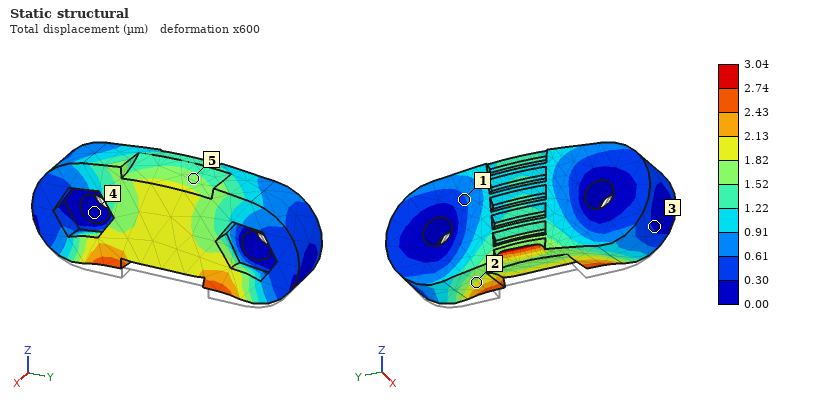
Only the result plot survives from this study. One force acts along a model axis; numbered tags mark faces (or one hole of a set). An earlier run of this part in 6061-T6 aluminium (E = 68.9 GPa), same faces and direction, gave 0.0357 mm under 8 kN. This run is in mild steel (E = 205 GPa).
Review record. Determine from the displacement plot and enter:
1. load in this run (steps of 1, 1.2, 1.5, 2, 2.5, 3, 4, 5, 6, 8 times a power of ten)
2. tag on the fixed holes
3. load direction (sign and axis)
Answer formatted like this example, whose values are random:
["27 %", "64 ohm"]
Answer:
["2 kN", "4", "+Z"]
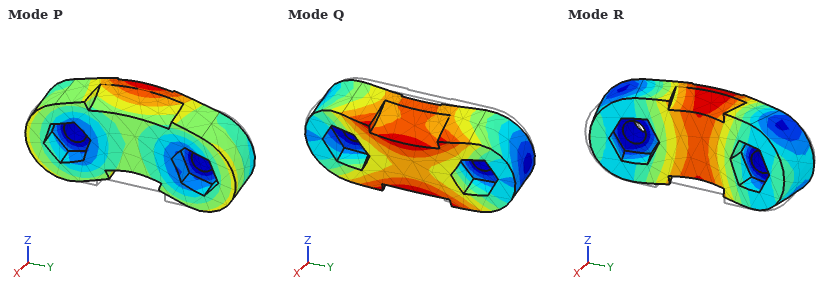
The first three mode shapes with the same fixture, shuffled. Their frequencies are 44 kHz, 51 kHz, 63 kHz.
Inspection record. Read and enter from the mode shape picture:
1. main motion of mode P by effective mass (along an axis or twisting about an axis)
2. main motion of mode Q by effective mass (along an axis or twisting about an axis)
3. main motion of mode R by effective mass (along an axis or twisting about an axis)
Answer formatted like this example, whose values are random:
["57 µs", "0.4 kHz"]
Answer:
["along Z", "along Z", "along X"]
